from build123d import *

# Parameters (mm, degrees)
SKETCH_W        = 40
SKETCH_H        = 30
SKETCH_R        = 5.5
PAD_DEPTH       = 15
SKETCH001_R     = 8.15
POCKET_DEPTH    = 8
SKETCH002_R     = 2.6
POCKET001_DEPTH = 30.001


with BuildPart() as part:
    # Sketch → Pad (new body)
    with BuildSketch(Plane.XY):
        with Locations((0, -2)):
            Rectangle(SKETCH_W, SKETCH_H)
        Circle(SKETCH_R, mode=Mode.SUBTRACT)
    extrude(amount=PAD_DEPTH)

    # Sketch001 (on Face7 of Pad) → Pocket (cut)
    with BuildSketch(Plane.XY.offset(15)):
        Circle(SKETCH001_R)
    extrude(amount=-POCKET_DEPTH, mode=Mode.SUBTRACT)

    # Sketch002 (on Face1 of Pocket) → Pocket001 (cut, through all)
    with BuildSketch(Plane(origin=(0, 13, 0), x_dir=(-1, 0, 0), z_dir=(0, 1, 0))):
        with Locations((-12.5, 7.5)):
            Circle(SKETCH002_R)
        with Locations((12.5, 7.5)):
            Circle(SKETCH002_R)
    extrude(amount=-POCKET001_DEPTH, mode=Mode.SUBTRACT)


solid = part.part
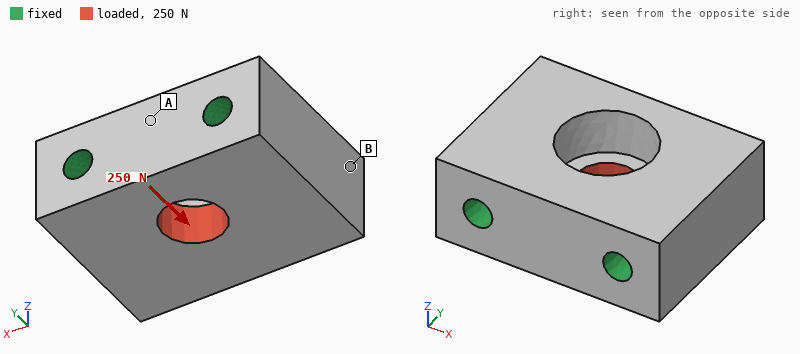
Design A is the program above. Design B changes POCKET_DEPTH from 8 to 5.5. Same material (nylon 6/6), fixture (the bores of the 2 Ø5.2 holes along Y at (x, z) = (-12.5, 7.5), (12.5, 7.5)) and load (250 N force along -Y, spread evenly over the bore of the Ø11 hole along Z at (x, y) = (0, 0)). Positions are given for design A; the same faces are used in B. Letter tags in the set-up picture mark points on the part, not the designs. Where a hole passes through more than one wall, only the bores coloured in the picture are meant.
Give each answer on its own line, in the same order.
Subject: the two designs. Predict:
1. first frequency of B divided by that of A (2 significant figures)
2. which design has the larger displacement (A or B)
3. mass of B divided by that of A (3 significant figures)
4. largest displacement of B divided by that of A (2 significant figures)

0.99
A
1.02
0.77
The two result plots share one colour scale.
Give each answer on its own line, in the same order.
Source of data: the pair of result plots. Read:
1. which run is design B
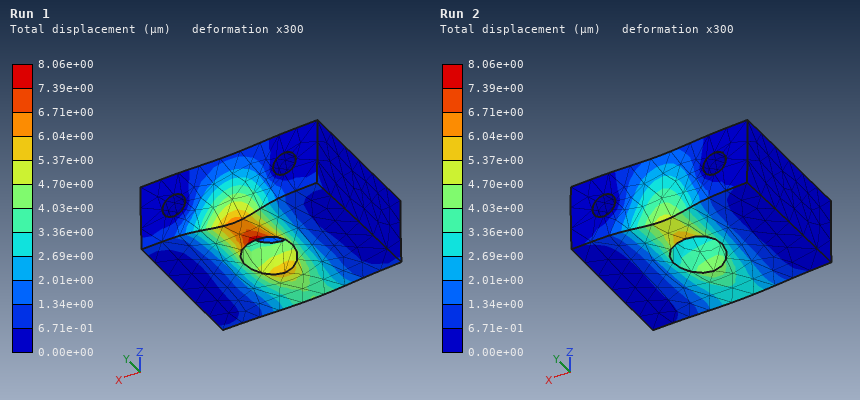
Run 2
